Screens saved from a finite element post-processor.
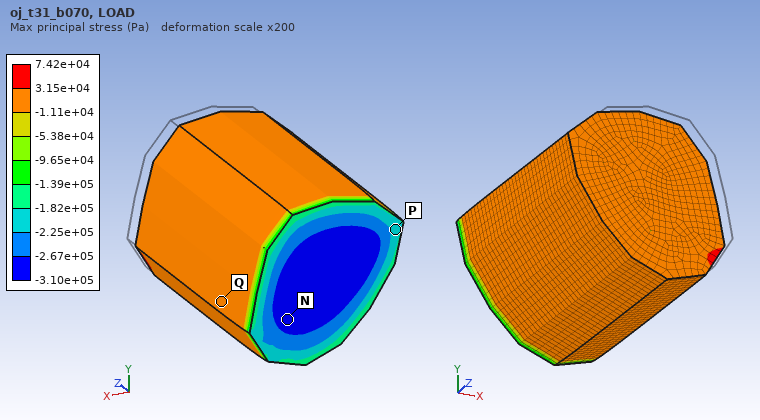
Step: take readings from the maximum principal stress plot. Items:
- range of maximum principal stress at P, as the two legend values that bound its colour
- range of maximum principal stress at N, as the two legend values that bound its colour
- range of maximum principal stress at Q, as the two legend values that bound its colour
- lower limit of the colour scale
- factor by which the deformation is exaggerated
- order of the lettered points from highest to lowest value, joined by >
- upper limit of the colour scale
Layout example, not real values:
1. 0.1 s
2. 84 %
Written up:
1. -2.25e+05 to -1.82e+05 Pa
2. -3.10e+05 to -2.67e+05 Pa
3. -1.11e+04 to 3.15e+04 Pa
4. -3.10e+05 Pa
5. 200
6. Q > P > N
7. 7.42e+04 Pa
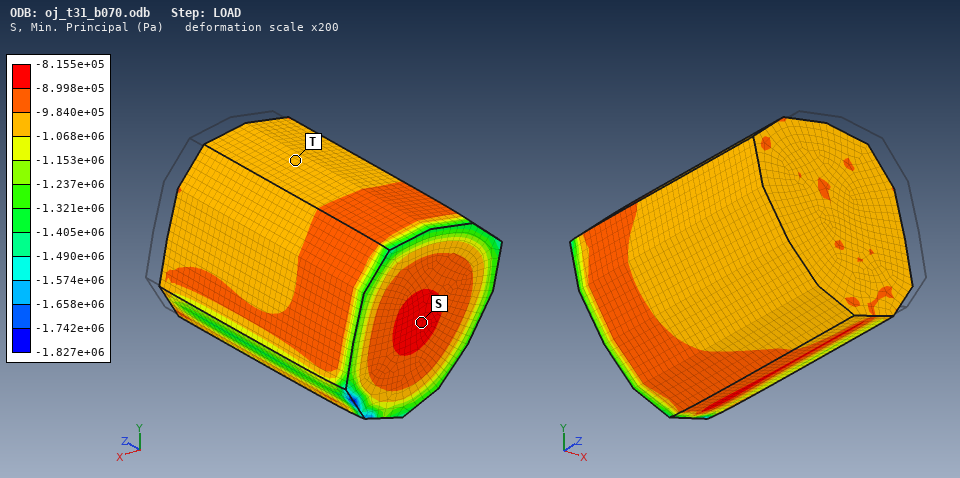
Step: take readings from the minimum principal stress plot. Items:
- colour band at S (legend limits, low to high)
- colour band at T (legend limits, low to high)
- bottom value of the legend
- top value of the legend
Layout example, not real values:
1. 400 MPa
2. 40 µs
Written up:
1. -8.998e+05 to -8.155e+05 Pa
2. -1.068e+06 to -9.840e+05 Pa
3. -1.827e+06 Pa
4. -8.155e+05 Pa
